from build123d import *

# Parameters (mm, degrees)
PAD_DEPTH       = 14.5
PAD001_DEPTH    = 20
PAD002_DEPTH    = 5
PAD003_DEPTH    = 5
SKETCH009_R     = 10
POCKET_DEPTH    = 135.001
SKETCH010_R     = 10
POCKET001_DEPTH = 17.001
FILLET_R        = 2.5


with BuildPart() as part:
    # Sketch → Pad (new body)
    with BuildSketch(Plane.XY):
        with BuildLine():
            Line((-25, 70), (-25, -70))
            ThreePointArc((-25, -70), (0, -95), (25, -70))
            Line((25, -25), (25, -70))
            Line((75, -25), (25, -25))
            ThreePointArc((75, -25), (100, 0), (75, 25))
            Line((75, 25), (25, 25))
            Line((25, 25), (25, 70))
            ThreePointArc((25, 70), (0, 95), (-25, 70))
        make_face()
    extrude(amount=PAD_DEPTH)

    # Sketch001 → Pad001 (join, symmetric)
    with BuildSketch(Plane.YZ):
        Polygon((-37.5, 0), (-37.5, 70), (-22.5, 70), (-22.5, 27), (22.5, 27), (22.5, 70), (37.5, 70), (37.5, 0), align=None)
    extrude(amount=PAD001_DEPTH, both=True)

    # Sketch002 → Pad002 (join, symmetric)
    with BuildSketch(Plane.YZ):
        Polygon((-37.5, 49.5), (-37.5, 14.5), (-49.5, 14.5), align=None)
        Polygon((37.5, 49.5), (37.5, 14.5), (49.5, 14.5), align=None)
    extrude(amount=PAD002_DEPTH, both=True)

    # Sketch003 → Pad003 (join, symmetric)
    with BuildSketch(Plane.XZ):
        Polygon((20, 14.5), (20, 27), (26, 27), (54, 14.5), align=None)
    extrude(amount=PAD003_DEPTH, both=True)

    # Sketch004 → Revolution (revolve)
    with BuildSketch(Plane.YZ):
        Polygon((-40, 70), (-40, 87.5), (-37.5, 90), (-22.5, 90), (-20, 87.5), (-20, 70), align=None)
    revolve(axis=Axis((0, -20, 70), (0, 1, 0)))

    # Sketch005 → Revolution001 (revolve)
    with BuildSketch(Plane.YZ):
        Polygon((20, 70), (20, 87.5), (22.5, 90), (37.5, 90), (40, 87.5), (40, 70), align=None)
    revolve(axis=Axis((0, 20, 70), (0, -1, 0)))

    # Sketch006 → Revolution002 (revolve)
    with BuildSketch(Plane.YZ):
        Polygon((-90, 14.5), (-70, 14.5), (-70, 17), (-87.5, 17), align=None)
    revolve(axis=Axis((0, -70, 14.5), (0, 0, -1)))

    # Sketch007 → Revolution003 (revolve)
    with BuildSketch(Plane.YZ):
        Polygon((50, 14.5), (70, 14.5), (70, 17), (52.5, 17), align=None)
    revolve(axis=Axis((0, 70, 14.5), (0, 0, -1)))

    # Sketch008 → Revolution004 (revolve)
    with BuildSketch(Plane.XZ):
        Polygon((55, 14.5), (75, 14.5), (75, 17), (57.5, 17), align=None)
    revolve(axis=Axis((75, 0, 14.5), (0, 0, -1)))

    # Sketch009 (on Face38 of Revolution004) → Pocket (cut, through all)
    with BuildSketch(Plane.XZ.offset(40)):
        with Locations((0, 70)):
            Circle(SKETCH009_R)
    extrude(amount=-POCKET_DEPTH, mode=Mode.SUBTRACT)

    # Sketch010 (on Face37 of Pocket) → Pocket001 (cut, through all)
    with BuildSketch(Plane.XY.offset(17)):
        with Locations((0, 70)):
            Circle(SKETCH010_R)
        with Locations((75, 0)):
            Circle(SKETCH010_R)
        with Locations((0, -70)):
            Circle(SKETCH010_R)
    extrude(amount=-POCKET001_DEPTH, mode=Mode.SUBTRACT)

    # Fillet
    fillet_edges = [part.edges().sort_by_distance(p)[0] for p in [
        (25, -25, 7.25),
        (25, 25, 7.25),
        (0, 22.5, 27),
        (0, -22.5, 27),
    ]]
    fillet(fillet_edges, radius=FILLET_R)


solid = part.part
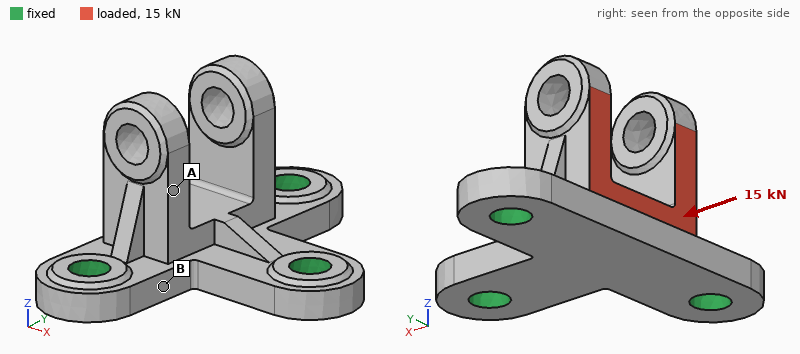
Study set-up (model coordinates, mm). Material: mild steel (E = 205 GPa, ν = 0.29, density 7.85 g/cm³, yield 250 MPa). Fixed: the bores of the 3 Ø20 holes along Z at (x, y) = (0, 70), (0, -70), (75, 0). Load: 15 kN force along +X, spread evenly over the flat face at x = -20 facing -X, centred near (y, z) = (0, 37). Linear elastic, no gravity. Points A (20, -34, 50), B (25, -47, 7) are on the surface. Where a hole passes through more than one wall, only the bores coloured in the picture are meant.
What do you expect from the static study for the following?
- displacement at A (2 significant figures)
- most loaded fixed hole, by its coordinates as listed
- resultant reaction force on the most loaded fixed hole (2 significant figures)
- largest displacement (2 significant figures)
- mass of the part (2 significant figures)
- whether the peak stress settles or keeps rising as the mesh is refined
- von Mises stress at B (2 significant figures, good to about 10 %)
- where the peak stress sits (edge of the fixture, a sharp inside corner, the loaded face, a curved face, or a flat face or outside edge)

35 µm
(75, 0)
10.0 kN
65 µm
2.2 kg
keeps rising
30 MPa
edge of the fixture
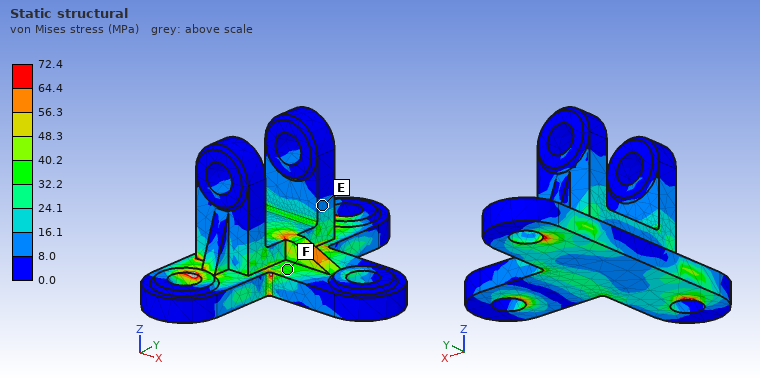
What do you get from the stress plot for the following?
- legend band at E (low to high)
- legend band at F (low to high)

8.0 to 16.1 MPa
32.2 to 40.2 MPa
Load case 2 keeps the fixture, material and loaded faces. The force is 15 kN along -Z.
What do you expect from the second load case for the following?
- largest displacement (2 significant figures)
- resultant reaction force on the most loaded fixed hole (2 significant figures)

68 µm
9.2 kN
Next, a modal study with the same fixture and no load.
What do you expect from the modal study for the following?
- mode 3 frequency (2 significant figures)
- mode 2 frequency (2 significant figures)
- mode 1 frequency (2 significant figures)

3100 Hz
3100 Hz
2600 Hz
